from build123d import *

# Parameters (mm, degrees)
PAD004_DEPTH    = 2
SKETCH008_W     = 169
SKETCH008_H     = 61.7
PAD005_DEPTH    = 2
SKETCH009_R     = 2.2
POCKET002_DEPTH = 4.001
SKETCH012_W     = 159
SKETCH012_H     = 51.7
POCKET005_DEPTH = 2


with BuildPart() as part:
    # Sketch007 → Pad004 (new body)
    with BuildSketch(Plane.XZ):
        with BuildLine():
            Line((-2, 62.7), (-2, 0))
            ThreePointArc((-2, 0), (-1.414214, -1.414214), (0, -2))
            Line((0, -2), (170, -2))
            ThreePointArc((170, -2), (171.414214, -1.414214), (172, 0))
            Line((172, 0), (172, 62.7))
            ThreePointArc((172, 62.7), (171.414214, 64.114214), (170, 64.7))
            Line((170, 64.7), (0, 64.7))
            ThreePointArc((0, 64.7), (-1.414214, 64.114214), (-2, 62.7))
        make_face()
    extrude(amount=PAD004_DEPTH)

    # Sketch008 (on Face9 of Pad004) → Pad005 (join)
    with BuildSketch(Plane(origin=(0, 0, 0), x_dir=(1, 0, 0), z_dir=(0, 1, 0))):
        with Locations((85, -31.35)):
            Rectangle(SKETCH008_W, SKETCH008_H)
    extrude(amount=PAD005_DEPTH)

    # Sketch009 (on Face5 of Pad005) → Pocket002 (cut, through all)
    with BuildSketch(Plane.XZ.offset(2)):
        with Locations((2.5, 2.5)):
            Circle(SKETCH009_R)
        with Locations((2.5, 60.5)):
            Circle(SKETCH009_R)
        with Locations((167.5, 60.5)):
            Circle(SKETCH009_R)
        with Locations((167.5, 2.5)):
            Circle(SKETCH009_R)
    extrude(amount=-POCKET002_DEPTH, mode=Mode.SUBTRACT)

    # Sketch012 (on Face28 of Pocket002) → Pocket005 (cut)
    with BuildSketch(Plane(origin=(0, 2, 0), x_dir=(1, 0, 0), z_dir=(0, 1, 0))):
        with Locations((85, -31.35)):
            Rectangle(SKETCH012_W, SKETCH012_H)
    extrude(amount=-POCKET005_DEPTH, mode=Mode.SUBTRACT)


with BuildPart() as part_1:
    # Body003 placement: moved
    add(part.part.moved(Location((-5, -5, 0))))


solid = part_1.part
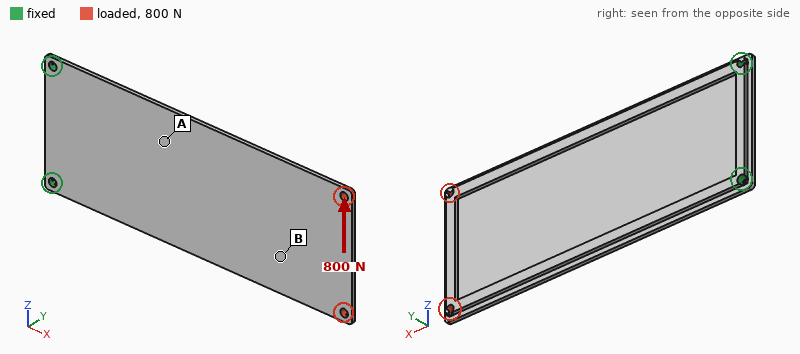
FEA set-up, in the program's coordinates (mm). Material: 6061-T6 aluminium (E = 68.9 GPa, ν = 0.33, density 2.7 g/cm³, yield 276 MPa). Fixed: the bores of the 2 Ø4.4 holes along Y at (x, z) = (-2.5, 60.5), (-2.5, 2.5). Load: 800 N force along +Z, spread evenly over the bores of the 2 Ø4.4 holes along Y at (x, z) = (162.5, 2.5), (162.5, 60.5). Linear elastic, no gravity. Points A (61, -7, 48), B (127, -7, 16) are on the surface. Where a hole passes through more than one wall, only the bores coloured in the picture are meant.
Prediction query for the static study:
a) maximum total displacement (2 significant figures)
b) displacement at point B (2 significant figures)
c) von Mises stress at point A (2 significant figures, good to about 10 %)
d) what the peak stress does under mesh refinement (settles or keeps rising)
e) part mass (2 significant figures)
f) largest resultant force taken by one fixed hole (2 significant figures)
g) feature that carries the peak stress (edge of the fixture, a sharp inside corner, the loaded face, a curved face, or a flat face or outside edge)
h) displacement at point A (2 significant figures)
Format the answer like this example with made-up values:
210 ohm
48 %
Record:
0.72 mm
0.30 mm
21 MPa
keeps rising
74 g
2.3 kN
a sharp inside corner
0.12 mm
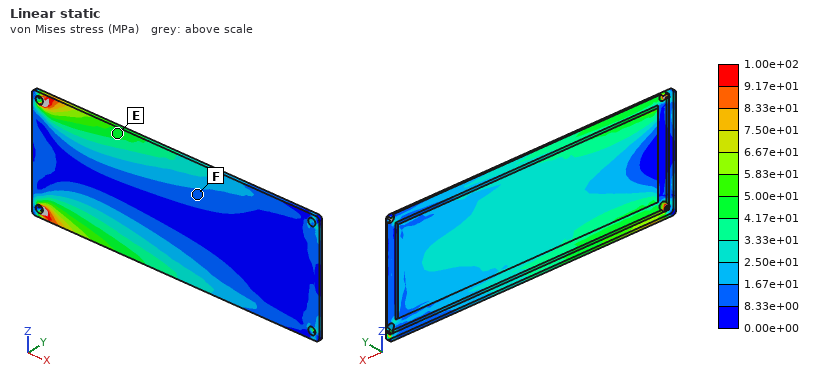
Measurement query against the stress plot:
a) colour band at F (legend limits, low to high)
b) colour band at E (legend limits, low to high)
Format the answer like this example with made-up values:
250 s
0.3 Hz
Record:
8.33e+00 to 1.67e+01 MPa
4.17e+01 to 5.00e+01 MPa
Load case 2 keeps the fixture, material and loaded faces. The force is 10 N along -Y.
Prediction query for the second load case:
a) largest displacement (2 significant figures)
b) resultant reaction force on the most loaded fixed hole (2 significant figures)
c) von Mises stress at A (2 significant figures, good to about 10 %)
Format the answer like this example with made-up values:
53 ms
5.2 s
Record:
1.9 mm
49 N
10 MPa
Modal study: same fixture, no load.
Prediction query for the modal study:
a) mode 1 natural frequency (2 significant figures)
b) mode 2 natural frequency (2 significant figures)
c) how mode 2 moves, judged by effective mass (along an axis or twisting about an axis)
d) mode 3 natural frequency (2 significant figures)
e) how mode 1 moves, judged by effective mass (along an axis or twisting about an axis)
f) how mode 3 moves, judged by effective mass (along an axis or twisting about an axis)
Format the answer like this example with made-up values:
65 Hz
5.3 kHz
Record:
84 Hz
360 Hz
twisting about X
530 Hz
along Y
along Y
